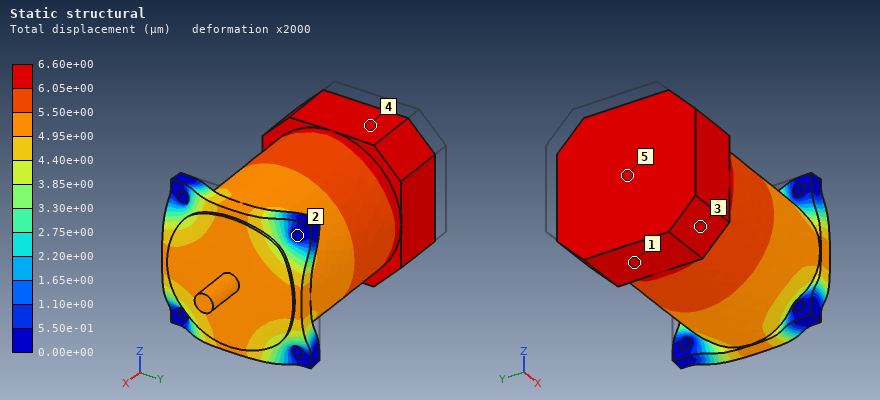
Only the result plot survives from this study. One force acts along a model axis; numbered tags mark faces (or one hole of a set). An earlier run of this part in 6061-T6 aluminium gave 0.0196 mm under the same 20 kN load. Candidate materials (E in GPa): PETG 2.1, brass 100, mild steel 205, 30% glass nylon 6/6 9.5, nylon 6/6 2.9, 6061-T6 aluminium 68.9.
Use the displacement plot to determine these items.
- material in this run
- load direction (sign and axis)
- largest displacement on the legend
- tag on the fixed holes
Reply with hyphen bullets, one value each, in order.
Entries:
- mild steel
- +X
- 6.60e+00 µm
- 2
